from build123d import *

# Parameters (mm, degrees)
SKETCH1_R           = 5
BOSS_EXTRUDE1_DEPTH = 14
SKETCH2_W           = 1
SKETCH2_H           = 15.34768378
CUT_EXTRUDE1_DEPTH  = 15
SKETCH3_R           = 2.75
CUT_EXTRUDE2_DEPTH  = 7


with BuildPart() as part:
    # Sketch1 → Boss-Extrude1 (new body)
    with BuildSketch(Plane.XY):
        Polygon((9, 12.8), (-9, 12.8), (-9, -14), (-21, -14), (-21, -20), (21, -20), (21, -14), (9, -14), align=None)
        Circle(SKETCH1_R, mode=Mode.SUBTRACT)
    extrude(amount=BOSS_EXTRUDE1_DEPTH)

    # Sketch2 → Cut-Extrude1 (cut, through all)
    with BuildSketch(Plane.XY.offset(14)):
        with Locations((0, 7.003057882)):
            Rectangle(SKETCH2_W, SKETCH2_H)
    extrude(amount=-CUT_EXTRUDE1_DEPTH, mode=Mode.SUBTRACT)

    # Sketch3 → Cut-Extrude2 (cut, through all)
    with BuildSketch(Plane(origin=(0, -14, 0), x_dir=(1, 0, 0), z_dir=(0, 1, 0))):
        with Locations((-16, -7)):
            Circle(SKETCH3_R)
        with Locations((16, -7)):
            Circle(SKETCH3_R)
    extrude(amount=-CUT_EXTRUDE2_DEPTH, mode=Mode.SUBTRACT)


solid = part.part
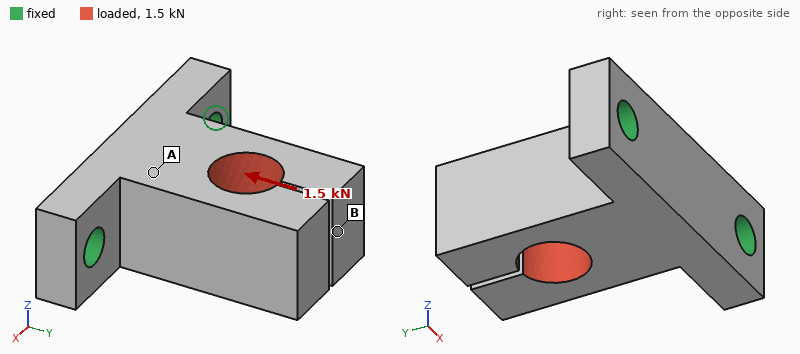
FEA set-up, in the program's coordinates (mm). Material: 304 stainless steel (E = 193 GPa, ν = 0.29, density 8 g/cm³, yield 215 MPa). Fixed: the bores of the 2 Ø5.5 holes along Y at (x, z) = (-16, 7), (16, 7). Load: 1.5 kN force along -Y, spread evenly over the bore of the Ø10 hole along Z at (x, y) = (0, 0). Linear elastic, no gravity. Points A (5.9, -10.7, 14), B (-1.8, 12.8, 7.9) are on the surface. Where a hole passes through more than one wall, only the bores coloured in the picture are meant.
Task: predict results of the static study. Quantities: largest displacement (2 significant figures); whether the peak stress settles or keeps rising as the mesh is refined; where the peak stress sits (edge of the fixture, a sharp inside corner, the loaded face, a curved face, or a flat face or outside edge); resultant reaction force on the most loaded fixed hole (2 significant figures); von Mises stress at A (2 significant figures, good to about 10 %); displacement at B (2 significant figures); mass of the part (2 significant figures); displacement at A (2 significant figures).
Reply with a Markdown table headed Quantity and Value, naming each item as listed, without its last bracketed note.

| Quantity | Value |
|---|---|
| largest displacement | 11 µm |
| whether the peak stress settles or keeps rising as the mesh is refined | keeps rising |
| where the peak stress sits | edge of the fixture |
| resultant reaction force on the most loaded fixed hole | 800 N |
| von Mises stress at A | 12 MPa |
| displacement at B | 11 µm |
| mass of the part | 70 g |
| displacement at A | 2.0 µm |
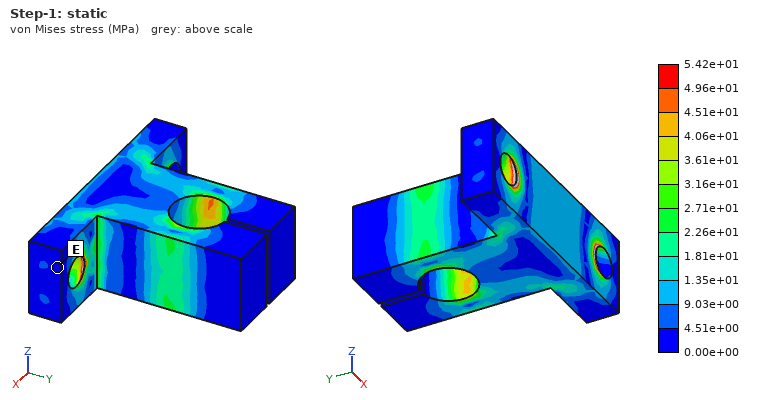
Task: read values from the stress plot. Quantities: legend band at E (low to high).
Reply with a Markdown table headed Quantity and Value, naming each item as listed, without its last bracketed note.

| Quantity | Value |
|---|---|
| legend band at E | 0.00e+00 to 4.51e+00 MPa |
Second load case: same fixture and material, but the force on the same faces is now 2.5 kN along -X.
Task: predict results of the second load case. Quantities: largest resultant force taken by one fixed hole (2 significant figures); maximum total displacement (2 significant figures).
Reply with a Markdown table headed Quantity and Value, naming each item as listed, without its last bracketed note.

| Quantity | Value |
|---|---|
| largest resultant force taken by one fixed hole | 2.2 kN |
| maximum total displacement | 38 µm |
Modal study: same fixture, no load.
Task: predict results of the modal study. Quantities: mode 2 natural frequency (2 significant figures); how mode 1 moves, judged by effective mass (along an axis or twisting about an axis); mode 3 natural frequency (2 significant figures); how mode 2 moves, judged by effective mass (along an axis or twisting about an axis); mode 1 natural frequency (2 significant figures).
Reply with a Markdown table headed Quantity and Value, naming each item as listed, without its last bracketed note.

| Quantity | Value |
|---|---|
| mode 2 natural frequency | 6300 Hz |
| how mode 1 moves, judged by effective mass | along Z |
| mode 3 natural frequency | 7000 Hz |
| how mode 2 moves, judged by effective mass | along X |
| mode 1 natural frequency | 4900 Hz |
